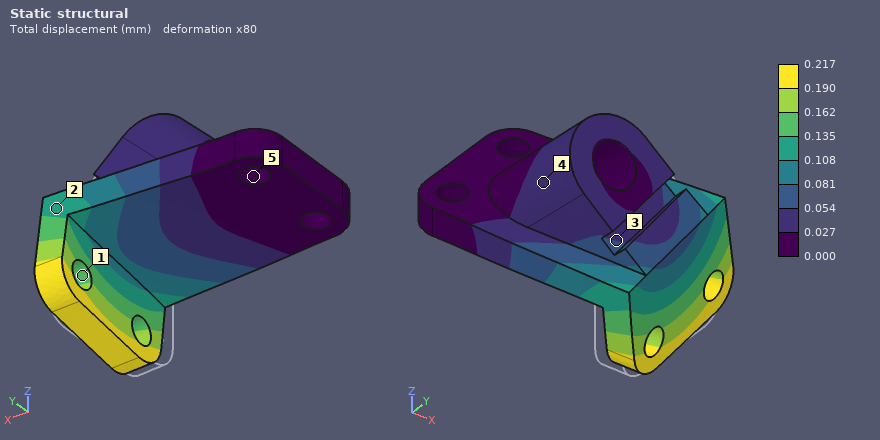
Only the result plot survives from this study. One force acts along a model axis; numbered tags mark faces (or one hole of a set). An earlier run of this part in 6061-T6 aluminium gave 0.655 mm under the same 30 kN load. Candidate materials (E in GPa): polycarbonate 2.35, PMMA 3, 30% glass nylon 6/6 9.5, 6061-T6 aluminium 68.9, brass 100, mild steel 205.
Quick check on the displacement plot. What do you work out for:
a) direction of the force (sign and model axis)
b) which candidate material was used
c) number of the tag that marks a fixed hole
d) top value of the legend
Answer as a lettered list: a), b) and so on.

a) +Y
b) mild steel
c) 5
d) 0.217 mm
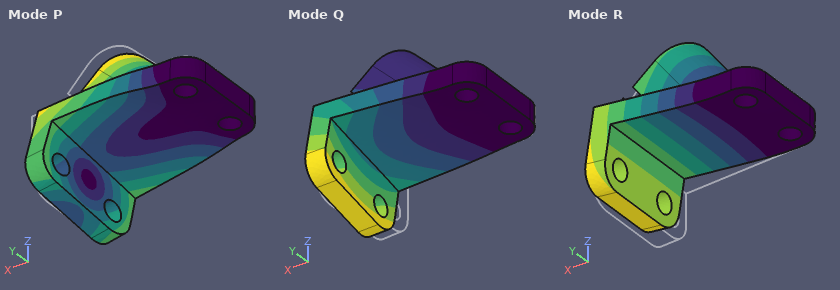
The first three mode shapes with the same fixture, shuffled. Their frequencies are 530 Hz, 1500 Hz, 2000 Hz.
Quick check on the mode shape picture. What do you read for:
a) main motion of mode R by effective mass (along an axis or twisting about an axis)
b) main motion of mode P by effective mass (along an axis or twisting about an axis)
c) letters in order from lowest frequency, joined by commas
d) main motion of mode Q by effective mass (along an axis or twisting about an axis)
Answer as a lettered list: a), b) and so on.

a) along Z
b) along Y
c) R, Q, P
d) along Y
